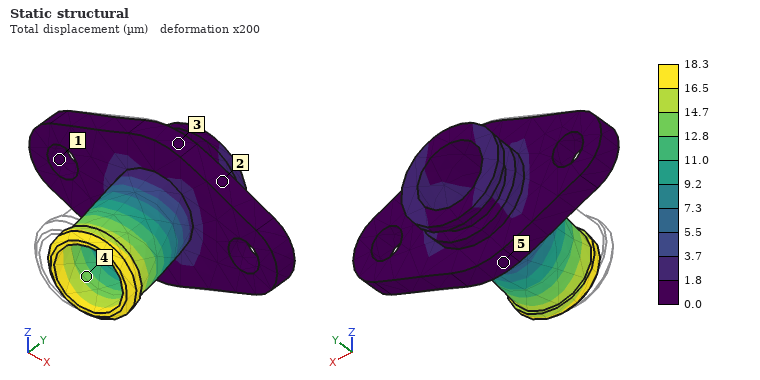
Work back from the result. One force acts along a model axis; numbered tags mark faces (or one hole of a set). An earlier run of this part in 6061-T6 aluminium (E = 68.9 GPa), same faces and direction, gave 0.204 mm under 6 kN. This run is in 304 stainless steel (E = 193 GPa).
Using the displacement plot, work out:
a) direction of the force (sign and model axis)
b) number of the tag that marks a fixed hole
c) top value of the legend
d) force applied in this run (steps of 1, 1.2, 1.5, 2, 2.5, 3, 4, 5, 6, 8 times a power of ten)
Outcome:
+X
1
18.3 µm
1.5 kN
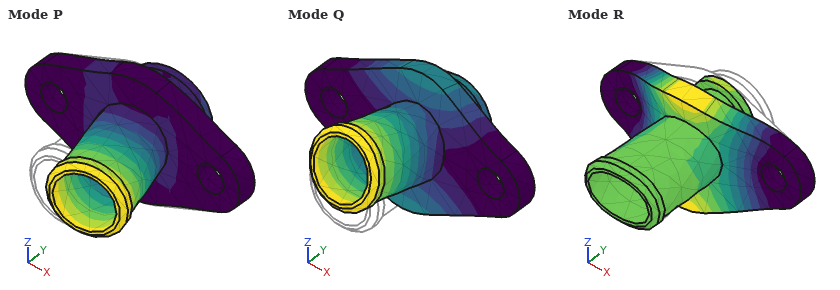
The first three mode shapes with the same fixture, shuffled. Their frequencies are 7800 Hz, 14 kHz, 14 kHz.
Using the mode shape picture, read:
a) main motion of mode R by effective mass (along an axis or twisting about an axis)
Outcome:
along Y
